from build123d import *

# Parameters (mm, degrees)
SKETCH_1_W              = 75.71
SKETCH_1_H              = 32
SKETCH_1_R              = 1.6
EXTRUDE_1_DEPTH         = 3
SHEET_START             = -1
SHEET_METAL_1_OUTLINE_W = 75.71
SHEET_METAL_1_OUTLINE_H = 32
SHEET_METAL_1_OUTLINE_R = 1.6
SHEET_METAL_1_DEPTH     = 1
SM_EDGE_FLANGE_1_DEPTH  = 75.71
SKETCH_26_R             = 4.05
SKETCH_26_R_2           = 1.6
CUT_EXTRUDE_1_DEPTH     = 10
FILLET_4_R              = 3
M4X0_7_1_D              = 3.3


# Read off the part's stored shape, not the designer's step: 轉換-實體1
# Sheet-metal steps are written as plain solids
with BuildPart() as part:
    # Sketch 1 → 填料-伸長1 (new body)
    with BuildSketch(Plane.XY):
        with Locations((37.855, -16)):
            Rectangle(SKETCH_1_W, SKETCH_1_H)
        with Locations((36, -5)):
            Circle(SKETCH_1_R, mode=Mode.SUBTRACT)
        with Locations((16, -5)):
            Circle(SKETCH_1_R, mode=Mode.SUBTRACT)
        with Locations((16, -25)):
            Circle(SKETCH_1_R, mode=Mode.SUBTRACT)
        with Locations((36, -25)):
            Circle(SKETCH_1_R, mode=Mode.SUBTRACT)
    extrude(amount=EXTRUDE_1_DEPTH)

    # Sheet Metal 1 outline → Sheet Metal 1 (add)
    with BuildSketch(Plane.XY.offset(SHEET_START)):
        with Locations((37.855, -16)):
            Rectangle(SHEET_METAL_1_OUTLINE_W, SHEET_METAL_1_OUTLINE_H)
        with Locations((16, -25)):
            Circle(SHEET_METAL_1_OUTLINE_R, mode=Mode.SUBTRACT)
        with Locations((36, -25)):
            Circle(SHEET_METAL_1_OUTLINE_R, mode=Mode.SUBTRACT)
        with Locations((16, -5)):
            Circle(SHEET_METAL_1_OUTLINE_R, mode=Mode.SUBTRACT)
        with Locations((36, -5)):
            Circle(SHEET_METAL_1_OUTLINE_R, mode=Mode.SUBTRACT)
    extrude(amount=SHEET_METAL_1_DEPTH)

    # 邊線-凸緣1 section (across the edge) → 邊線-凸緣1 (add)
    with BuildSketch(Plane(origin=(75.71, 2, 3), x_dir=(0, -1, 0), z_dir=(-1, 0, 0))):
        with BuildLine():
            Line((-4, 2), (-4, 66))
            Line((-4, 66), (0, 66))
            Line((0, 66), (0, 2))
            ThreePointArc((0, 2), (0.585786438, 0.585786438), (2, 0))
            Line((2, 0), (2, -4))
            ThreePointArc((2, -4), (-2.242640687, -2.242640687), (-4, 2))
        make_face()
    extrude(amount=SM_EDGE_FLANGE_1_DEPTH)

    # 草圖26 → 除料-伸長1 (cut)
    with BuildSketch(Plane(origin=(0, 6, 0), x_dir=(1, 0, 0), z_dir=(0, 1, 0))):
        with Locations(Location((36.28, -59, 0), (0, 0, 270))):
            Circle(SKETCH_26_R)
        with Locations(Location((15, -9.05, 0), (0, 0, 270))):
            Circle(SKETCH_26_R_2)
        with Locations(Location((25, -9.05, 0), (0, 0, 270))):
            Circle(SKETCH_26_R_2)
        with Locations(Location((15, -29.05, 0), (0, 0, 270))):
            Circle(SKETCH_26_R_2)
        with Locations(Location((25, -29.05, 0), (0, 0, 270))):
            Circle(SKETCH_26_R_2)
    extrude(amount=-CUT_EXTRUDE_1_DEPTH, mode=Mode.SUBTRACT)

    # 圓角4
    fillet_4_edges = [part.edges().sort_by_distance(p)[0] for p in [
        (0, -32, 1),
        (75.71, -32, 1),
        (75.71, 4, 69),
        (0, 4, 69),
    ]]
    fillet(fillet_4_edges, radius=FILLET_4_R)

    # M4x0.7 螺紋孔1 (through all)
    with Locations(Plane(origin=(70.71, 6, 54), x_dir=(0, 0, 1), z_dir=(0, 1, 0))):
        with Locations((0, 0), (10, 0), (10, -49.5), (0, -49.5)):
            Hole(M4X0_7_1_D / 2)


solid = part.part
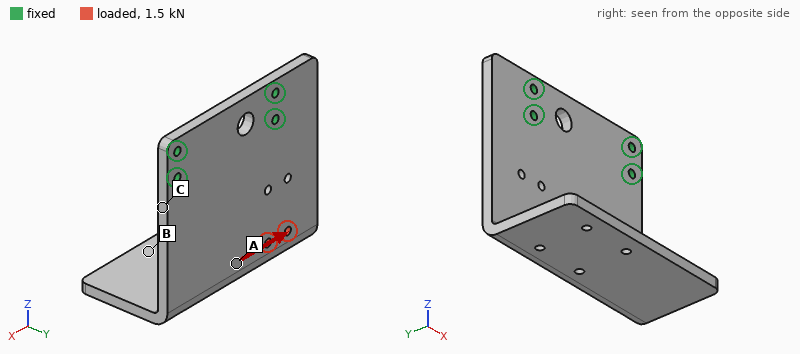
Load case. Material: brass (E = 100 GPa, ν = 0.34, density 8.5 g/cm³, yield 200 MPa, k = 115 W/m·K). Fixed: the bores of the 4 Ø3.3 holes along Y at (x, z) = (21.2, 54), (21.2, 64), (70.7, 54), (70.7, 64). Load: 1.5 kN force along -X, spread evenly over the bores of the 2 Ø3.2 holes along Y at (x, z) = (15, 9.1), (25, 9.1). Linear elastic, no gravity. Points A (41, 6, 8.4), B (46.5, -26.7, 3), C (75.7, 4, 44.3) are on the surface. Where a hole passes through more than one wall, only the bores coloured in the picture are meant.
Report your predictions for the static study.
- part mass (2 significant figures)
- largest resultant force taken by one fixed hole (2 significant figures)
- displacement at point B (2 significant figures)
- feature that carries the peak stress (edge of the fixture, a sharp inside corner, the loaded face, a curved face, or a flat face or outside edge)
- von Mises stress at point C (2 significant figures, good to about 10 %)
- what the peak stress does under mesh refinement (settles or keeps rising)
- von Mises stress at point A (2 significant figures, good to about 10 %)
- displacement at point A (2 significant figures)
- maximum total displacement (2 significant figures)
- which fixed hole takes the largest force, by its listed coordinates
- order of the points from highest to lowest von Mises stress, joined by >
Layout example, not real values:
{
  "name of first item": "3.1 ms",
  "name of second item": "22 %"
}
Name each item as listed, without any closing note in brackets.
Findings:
{
  "part mass": "260 g",
  "largest resultant force taken by one fixed hole": "1.3 kN",
  "displacement at point B": "15 µm",
  "feature that carries the peak stress": "edge of the fixture",
  "von Mises stress at point C": "18 MPa",
  "what the peak stress does under mesh refinement": "keeps rising",
  "von Mises stress at point A": "10 MPa",
  "displacement at point A": "14 µm",
  "maximum total displacement": "20 µm",
  "which fixed hole takes the largest force, by its listed coordinates": "(21.2, 54)",
  "order of the points from highest to lowest von Mises stress, joined by >": "C > A > B"
}
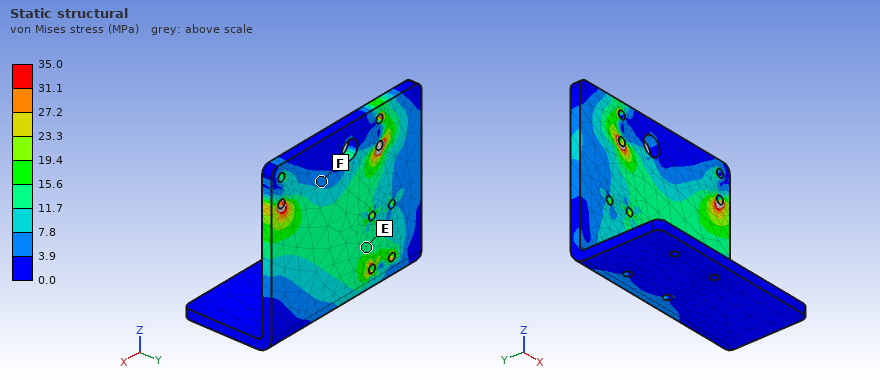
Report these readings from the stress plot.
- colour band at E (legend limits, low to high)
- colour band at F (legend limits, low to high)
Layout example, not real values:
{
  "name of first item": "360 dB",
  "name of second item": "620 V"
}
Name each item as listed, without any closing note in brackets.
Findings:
{
  "colour band at E": "11.7 to 15.6 MPa",
  "colour band at F": "3.9 to 7.8 MPa"
}
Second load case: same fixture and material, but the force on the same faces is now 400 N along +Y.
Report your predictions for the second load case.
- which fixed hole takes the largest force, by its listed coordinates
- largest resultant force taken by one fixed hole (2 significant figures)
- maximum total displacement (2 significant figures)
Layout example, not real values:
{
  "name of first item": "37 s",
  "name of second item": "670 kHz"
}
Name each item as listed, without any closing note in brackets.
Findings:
{
  "which fixed hole takes the largest force, by its listed coordinates": "(21.2, 54)",
  "largest resultant force taken by one fixed hole": "990 N",
  "maximum total displacement": "0.73 mm"
}
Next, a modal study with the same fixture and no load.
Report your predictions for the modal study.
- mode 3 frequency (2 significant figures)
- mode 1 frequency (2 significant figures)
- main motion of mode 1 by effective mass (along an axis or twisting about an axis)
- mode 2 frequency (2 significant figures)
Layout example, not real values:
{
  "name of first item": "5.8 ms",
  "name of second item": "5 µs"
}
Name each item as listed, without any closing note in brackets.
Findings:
{
  "mode 3 frequency": "1200 Hz",
  "mode 1 frequency": "340 Hz",
  "main motion of mode 1 by effective mass": "along Y",
  "mode 2 frequency": "680 Hz"
}
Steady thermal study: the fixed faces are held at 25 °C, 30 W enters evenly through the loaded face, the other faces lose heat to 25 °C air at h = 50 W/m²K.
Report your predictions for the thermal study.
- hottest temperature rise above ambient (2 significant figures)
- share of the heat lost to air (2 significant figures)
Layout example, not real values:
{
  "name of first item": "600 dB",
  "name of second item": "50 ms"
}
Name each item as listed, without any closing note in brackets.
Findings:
{
  "hottest temperature rise above ambient": "44 K",
  "share of the heat lost to air": "47 %"
}
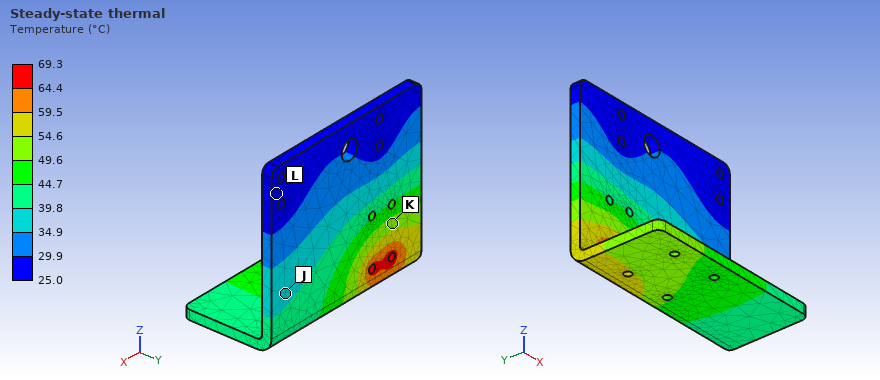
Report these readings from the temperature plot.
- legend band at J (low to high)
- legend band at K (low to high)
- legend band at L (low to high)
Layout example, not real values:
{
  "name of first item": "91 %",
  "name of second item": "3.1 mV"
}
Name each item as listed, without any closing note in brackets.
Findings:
{
  "legend band at J": "34.9 to 39.8 °C",
  "legend band at K": "49.6 to 54.6 °C",
  "legend band at L": "25.0 to 29.9 °C"
}
